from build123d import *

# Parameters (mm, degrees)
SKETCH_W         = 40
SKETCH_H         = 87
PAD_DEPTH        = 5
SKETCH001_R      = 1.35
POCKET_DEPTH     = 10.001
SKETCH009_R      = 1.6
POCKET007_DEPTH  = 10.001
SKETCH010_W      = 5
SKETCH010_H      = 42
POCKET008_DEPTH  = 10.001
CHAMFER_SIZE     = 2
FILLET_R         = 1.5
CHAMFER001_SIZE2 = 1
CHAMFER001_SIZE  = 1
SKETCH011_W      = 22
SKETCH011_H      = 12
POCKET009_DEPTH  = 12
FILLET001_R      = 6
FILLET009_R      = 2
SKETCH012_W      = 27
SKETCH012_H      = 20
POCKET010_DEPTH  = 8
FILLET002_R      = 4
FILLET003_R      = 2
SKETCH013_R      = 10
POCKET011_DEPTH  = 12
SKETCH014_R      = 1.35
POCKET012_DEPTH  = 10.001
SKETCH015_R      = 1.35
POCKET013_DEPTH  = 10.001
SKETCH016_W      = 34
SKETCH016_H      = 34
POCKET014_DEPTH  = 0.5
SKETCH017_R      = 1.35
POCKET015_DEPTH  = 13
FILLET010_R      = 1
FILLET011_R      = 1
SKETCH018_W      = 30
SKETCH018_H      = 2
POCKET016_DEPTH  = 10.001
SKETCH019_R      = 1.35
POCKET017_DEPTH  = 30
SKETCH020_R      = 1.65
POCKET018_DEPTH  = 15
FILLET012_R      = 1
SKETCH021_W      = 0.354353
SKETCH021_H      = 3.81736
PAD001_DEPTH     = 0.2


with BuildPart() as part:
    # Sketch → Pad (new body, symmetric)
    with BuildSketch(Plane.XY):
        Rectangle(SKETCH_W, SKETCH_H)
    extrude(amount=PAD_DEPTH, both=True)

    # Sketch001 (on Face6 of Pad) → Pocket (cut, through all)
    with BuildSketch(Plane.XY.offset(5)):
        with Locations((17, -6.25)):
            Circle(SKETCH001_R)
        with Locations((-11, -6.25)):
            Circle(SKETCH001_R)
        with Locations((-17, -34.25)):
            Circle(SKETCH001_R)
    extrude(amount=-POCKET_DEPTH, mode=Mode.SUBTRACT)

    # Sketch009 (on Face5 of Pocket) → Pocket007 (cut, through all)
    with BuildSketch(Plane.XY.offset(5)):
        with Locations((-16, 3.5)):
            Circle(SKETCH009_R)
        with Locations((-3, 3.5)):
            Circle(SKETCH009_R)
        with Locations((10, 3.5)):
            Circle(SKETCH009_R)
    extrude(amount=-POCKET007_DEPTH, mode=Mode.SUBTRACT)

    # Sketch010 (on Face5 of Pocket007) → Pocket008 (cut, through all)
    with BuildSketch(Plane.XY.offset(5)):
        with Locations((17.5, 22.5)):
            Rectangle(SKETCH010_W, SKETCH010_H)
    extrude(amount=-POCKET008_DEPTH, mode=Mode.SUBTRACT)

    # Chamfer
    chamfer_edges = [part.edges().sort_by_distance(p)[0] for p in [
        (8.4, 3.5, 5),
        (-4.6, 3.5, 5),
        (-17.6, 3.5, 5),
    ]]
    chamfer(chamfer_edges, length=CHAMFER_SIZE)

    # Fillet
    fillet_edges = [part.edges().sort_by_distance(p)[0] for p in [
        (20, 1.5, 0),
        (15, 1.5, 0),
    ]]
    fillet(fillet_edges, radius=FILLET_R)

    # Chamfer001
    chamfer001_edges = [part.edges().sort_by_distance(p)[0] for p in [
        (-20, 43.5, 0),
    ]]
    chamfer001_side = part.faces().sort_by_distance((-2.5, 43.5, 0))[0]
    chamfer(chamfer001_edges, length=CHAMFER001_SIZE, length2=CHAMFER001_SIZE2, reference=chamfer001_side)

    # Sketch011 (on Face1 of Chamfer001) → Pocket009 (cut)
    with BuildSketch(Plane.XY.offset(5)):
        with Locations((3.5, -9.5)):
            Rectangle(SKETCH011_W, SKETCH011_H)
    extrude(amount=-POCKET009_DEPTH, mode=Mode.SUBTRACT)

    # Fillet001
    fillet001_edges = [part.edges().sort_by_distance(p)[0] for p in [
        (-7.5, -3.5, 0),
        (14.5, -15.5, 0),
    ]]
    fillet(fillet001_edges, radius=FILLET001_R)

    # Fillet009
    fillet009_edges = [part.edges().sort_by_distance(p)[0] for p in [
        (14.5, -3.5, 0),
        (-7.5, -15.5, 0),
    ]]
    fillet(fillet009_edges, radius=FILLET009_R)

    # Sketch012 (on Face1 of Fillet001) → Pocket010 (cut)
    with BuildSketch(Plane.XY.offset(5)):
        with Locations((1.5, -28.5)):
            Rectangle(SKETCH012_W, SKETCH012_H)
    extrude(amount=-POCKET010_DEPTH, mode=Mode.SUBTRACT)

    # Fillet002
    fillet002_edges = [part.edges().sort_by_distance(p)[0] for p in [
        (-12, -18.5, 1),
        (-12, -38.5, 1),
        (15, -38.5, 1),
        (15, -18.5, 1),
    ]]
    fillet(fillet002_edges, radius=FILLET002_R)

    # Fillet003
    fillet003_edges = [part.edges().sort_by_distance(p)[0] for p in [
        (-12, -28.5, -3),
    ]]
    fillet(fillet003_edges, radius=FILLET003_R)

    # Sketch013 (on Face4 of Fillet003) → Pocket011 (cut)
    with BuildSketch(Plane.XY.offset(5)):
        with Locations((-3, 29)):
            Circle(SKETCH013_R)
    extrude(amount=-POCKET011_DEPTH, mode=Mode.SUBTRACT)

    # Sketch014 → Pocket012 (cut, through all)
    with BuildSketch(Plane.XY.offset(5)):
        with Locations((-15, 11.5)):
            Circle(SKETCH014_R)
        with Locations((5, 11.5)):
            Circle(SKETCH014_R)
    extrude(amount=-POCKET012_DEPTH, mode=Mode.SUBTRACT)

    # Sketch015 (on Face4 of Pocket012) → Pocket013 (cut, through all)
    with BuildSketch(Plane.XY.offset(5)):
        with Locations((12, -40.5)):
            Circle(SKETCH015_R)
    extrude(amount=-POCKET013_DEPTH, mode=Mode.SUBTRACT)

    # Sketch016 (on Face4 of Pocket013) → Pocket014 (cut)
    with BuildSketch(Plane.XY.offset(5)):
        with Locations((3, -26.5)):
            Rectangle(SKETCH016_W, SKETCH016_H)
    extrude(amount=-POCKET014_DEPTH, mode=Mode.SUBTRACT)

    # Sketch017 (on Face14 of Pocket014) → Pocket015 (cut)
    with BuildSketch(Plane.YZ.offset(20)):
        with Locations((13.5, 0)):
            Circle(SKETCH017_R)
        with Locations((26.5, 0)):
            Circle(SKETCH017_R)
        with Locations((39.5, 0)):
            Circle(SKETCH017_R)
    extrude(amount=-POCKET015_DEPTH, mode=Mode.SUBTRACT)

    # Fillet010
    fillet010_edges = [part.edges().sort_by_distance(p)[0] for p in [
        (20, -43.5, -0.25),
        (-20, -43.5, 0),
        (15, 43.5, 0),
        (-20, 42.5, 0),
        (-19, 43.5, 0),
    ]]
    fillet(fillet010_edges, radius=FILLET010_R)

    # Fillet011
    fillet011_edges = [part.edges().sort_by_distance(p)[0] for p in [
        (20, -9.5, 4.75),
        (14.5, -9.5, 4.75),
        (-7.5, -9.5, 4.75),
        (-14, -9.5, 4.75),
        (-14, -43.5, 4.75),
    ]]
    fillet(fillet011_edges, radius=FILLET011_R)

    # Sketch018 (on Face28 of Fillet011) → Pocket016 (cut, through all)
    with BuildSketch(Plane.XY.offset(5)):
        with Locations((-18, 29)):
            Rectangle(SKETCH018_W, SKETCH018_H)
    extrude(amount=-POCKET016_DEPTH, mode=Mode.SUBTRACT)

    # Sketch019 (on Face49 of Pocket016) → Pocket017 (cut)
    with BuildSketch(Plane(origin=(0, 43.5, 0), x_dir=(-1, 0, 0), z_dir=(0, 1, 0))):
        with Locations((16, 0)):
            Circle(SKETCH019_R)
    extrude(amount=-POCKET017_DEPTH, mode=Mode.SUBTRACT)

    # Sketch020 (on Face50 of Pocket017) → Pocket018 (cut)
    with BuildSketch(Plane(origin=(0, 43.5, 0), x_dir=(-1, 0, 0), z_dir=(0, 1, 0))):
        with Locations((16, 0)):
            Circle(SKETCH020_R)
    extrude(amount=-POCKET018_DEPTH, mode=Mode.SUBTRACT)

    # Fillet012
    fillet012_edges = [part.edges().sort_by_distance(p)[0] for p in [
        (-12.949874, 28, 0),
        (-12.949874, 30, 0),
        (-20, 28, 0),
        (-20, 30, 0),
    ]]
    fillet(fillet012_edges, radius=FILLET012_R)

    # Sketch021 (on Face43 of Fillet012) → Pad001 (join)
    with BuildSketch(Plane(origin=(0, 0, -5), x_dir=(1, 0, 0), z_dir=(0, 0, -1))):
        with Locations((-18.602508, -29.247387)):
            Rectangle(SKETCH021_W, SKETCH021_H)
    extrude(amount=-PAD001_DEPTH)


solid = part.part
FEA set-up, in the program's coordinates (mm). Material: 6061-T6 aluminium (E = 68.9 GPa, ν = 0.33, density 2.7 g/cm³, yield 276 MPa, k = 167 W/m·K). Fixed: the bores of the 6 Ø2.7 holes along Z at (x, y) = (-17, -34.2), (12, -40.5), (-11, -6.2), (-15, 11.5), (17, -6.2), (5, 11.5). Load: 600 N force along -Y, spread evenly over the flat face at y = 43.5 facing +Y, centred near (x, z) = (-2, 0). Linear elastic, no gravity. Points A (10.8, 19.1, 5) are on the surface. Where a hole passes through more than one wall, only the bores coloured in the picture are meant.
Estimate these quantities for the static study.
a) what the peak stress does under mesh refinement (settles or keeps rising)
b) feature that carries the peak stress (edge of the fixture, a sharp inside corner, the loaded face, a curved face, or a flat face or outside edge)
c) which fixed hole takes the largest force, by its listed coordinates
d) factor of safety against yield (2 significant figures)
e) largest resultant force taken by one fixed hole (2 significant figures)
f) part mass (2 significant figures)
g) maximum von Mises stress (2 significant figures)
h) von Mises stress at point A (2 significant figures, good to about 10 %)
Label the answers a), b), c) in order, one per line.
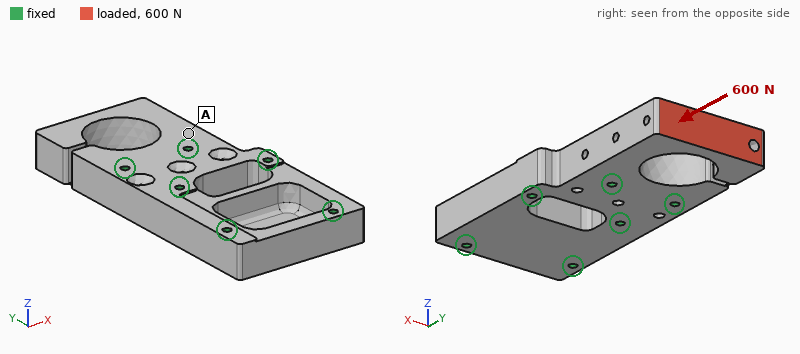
a) settles
b) a flat face or outside edge
c) (5, 11.5)
d) 0.14
e) 380 N
f) 58 g
g) 2000 MPa
h) 9.4 MPa
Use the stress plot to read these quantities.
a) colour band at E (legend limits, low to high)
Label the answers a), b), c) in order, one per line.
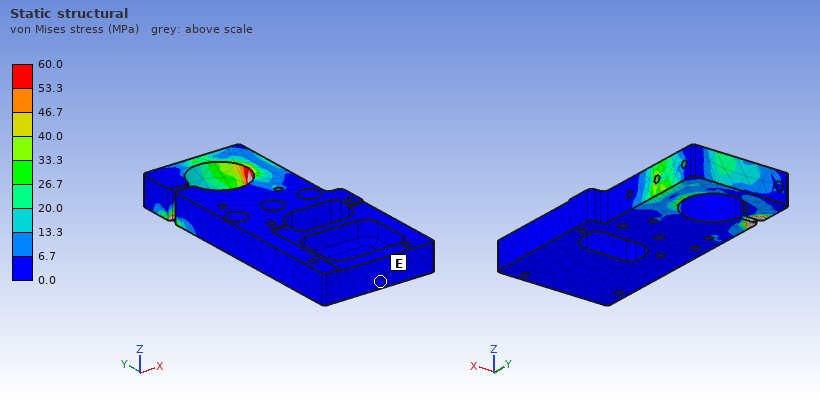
a) 0.0 to 6.7 MPa
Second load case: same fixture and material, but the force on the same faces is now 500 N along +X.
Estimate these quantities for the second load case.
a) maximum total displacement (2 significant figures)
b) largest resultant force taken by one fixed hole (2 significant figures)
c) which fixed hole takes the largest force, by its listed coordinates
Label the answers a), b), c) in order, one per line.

a) 89 µm
b) 500 N
c) (-15, 11.5)
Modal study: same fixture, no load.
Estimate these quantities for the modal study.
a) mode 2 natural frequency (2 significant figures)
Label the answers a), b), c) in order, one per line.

a) 4500 Hz
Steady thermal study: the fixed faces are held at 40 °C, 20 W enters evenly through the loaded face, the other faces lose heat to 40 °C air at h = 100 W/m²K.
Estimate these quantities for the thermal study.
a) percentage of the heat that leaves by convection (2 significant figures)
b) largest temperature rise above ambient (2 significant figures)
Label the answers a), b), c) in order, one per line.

a) 29 %
b) 41 K
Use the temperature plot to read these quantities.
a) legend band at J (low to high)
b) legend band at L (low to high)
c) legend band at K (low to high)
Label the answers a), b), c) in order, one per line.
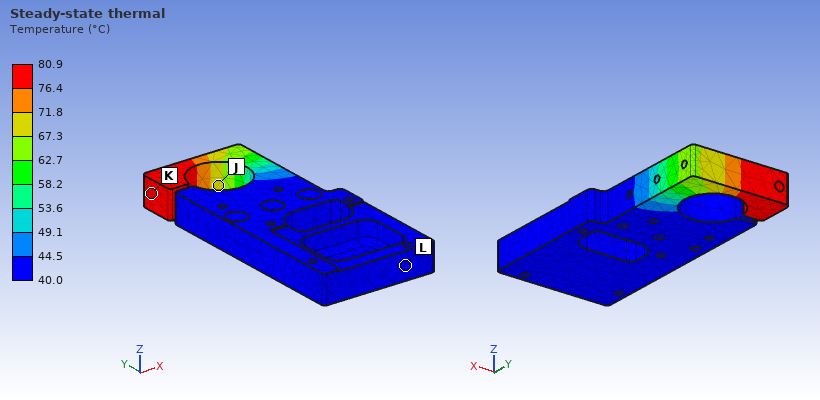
a) 67.3 to 71.8 °C
b) 40.0 to 44.5 °C
c) 76.4 to 80.9 °C
